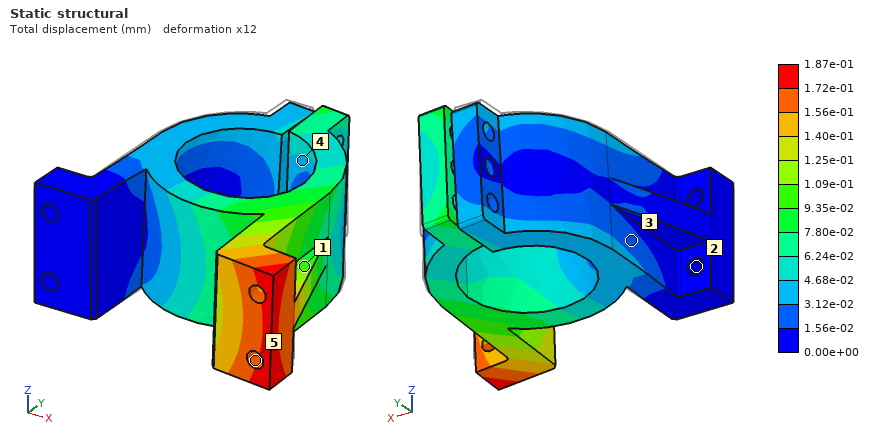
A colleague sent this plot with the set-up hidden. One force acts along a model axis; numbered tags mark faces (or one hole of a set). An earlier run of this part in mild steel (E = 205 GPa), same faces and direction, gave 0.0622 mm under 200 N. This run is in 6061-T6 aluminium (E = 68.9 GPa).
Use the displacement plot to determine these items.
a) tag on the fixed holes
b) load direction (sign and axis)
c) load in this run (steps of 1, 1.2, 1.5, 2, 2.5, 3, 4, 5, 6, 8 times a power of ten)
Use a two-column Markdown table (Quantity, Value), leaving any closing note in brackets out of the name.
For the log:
| Quantity | Value |
|---|---|
| tag on the fixed holes | 2 |
| load direction | -Z |
| load in this run | 200 N |
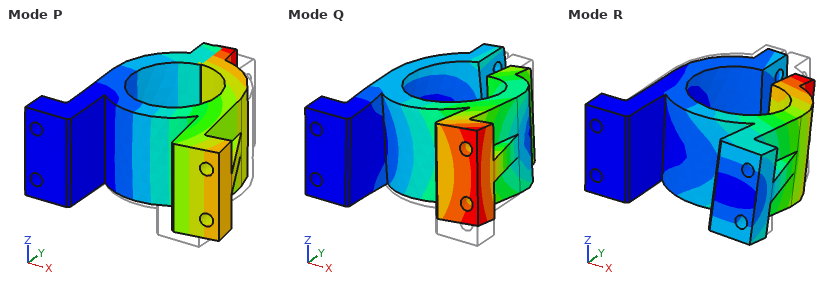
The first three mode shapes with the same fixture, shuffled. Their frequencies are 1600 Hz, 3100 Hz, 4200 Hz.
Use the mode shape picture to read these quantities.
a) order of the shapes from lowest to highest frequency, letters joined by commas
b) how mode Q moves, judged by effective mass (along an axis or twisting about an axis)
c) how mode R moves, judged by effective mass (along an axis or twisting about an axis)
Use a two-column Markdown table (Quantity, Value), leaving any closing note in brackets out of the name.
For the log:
| Quantity | Value |
|---|---|
| order of the shapes from lowest to highest frequency, letters joined by commas | P, R, Q |
| how mode Q moves, judged by effective mass | along Z |
| how mode R moves, judged by effective mass | along Z |
